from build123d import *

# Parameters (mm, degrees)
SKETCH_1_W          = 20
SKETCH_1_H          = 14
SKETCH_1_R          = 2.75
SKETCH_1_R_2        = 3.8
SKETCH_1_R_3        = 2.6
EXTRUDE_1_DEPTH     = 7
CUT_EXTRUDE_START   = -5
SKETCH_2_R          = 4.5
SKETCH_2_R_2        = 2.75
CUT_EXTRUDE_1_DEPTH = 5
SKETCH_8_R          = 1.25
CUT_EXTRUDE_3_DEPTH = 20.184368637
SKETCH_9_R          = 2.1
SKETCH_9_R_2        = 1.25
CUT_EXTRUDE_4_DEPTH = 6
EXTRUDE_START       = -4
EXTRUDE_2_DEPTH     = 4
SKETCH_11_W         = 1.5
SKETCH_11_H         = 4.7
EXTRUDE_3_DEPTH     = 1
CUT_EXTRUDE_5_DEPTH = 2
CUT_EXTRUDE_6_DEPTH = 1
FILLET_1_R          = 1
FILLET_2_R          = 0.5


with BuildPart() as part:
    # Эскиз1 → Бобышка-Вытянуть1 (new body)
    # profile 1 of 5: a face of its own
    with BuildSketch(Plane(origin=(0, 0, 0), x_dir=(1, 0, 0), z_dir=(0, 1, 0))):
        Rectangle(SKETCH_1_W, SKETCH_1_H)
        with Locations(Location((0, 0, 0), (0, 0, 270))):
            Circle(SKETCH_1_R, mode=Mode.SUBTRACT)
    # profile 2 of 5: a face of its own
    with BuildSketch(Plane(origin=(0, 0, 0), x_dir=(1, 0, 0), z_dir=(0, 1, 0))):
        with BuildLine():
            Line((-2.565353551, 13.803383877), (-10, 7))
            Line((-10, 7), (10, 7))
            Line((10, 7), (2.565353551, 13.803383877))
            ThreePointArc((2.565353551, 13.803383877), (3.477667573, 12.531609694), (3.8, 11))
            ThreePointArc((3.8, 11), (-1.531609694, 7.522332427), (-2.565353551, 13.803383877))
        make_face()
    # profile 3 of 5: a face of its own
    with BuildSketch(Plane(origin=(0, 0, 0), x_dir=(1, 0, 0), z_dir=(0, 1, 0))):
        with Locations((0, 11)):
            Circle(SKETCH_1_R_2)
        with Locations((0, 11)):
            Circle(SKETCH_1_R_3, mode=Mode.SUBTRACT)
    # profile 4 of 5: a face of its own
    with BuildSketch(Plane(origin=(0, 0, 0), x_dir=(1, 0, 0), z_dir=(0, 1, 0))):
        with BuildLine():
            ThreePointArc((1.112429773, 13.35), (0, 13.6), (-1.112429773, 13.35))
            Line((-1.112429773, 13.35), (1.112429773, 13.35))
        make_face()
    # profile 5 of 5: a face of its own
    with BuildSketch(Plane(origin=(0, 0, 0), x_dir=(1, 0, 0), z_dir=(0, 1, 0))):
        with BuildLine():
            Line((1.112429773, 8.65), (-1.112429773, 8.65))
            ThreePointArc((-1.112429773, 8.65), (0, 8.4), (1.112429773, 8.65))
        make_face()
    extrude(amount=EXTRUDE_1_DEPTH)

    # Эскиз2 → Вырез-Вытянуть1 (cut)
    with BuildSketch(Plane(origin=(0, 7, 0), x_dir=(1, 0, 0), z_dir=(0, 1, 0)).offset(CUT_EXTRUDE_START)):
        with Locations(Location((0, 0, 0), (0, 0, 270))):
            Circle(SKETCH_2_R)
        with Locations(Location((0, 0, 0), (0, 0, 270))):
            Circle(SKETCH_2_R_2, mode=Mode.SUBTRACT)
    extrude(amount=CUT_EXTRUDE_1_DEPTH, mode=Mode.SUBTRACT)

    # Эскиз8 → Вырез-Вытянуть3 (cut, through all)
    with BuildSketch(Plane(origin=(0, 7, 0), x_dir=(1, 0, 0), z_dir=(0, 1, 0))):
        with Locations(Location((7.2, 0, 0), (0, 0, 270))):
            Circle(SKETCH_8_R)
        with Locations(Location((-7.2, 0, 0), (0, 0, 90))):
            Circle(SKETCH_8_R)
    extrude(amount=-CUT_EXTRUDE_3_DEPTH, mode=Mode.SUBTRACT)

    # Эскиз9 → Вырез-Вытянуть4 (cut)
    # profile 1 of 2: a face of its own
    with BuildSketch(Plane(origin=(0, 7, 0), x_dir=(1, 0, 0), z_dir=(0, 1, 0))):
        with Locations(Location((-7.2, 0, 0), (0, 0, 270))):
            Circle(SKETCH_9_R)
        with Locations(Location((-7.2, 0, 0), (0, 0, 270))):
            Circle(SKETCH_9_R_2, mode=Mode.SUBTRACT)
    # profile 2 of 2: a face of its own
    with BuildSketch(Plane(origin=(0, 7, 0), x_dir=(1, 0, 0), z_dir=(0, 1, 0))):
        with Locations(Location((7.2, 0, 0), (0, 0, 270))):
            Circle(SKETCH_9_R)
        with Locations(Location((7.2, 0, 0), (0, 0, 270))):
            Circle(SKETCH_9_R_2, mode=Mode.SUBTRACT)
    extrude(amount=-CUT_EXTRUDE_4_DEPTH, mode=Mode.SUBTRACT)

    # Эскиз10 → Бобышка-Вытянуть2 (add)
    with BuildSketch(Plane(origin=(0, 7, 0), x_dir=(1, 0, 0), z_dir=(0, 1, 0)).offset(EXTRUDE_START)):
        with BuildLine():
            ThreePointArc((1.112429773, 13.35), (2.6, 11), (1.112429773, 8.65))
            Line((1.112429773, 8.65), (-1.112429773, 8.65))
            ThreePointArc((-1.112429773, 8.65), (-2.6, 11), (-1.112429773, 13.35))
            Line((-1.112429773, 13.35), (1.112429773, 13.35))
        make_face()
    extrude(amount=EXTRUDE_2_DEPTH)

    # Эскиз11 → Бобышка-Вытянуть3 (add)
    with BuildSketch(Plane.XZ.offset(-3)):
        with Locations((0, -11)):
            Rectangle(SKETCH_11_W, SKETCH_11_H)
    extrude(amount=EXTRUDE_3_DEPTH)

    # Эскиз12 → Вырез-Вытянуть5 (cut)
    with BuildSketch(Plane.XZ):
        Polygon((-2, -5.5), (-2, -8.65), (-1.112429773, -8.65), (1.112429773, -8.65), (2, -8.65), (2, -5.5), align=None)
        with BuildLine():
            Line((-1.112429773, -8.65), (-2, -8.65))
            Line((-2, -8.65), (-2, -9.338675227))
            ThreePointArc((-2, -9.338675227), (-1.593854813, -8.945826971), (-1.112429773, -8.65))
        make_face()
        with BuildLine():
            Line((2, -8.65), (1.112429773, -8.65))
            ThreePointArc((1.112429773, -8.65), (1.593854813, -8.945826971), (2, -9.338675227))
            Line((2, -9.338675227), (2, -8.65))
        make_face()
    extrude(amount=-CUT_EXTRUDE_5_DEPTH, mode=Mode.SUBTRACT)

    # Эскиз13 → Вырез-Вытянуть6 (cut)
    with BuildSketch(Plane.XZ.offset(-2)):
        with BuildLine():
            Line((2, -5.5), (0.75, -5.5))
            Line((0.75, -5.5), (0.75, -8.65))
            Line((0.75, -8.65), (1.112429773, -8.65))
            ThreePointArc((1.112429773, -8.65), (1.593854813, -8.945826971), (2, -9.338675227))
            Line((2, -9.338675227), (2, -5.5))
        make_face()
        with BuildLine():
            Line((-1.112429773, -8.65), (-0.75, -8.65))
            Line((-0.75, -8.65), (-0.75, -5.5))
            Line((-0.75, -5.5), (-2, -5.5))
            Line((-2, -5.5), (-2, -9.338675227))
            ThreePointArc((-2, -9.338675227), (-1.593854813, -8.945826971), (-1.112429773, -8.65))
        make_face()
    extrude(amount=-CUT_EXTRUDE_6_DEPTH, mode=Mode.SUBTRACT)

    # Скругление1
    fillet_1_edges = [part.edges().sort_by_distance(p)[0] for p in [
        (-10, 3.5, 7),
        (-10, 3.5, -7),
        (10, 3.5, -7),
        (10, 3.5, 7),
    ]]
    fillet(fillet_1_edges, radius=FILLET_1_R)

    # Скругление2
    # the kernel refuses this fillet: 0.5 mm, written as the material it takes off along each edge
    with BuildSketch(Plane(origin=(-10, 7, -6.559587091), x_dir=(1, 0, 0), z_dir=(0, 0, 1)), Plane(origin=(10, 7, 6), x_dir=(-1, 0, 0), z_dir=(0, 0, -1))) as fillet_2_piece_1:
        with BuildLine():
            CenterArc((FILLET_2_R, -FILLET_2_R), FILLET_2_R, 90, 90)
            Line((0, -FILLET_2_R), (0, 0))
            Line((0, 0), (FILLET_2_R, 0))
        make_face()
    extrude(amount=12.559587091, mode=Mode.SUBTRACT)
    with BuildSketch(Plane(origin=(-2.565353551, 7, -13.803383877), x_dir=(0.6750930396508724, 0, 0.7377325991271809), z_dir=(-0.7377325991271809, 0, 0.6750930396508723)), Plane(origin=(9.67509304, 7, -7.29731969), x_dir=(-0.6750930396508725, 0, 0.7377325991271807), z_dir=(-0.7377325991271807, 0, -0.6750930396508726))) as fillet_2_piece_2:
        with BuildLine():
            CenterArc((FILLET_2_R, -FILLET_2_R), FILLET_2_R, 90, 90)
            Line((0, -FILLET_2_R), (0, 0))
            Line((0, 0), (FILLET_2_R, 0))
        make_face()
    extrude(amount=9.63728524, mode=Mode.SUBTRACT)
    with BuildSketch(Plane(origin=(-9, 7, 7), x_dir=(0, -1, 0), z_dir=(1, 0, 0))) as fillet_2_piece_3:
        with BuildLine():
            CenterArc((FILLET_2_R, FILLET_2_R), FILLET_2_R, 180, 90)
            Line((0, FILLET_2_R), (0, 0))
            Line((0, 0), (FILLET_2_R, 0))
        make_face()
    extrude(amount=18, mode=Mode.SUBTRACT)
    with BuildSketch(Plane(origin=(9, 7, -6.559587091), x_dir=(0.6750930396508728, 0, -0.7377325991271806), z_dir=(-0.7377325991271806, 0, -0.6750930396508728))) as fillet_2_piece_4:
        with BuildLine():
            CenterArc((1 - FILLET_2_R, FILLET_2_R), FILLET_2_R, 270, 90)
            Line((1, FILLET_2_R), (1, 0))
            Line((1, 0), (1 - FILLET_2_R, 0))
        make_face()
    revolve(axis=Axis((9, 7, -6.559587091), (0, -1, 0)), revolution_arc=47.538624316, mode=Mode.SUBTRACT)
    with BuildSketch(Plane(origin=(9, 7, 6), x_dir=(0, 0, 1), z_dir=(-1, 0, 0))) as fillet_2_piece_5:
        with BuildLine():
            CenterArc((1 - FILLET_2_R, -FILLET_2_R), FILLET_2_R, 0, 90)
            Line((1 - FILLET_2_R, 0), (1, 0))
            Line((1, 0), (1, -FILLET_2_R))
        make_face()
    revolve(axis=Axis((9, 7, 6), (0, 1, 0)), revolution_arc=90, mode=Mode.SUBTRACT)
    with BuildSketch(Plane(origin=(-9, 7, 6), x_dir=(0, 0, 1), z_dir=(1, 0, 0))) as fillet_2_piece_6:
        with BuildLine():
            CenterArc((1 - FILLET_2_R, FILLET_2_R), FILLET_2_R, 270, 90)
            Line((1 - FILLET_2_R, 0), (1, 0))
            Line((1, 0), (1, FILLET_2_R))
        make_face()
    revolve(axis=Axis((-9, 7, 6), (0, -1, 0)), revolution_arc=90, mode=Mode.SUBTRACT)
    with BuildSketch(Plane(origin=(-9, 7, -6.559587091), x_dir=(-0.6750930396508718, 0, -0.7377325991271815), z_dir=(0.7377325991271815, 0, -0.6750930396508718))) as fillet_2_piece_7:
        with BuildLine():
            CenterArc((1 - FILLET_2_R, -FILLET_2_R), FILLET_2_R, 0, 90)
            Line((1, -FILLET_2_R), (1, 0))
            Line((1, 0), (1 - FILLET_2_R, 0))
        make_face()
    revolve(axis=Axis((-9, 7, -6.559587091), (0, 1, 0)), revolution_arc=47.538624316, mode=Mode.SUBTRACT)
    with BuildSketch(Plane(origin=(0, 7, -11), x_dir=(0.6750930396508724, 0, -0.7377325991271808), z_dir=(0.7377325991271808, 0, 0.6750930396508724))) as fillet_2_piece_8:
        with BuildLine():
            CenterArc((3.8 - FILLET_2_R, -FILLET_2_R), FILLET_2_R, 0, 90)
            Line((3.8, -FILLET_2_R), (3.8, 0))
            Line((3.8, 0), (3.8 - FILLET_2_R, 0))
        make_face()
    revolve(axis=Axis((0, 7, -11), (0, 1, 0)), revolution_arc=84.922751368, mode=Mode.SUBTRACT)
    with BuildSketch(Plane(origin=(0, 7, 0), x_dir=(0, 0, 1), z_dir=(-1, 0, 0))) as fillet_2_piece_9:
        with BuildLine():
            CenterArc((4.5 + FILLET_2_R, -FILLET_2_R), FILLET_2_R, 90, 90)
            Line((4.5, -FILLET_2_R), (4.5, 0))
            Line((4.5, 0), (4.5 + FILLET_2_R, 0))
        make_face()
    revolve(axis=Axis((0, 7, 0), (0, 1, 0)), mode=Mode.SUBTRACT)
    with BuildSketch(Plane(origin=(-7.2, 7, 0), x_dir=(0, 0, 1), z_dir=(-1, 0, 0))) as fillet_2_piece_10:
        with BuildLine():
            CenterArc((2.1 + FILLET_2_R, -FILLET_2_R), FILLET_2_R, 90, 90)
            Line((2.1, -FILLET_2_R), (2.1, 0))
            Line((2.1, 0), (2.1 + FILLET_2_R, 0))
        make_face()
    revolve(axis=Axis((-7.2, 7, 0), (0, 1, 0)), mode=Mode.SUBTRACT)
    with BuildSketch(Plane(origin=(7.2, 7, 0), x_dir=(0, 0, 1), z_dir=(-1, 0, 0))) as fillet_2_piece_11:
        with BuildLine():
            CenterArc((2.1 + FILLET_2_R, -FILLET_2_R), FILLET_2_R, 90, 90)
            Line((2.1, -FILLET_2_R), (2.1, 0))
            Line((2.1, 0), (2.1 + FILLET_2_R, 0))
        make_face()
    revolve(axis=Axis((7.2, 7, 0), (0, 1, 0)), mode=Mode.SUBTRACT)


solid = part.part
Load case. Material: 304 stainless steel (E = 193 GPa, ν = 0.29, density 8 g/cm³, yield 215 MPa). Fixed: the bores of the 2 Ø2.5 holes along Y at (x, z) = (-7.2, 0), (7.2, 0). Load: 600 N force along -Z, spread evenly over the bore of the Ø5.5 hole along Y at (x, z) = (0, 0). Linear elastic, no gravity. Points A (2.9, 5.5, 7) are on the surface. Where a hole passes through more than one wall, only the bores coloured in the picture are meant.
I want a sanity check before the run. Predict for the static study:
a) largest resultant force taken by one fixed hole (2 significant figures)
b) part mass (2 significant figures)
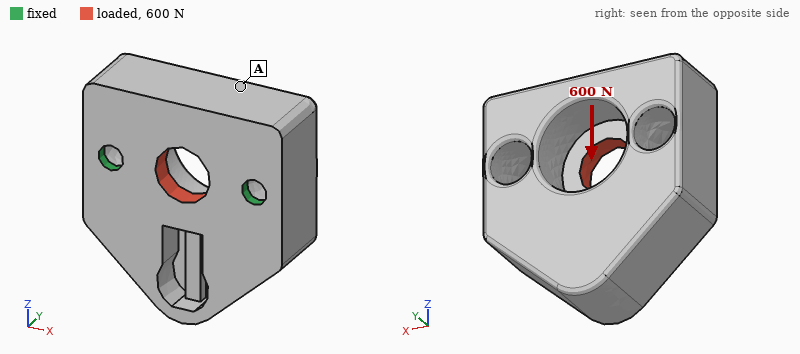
300 N
16 g
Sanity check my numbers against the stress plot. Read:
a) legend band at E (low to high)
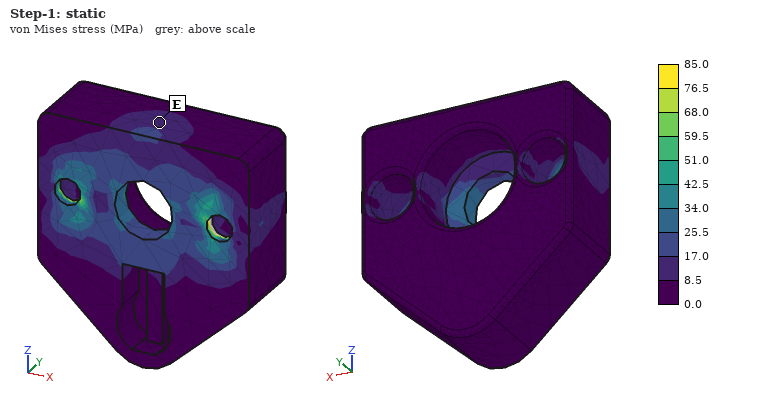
8.5 to 17.0 MPa
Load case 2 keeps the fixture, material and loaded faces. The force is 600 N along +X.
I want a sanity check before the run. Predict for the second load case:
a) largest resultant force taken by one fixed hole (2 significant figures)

300 N
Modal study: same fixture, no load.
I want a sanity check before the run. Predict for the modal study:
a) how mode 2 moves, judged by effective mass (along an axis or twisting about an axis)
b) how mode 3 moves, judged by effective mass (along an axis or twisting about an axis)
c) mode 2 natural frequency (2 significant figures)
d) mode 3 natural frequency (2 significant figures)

along X
along Y
25 kHz
27 kHz
